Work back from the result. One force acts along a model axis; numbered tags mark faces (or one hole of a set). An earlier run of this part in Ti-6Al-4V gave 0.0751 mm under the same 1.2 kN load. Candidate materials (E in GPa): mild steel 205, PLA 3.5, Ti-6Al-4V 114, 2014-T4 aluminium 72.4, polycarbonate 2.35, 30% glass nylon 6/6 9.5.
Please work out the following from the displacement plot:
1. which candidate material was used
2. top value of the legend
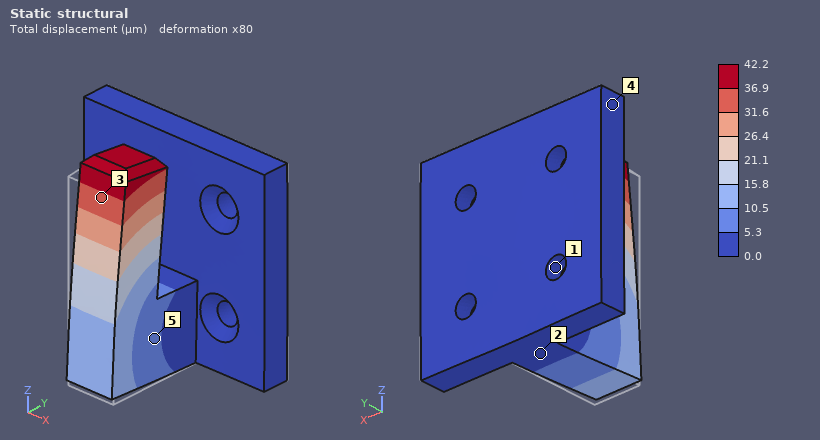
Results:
mild steel
42.2 µm
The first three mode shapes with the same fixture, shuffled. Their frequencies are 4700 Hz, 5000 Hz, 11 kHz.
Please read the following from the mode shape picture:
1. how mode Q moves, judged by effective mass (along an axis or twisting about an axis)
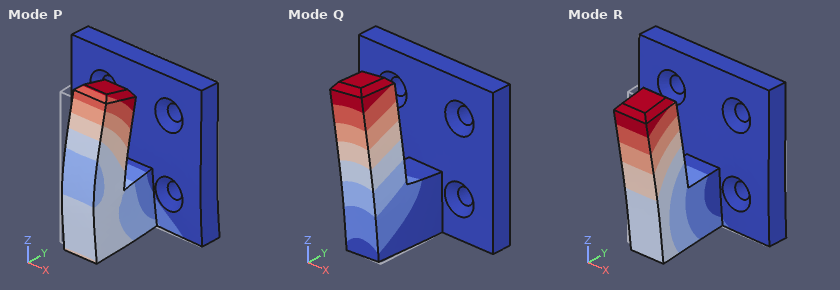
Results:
along X
